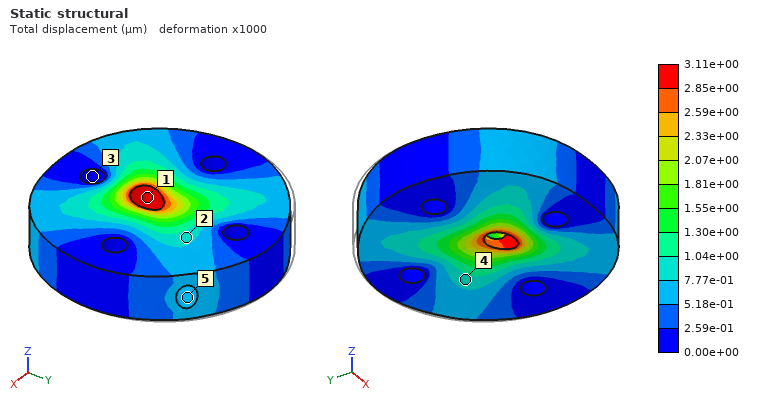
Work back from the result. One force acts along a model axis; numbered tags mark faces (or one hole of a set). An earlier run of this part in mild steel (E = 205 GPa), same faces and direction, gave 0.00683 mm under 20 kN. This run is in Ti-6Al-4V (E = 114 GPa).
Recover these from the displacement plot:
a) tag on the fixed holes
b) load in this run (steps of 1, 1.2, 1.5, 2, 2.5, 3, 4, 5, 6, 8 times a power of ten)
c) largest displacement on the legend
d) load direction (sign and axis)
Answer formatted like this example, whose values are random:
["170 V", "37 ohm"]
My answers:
["3", "5 kN", "3.11e+00 µm", "-Y"]
